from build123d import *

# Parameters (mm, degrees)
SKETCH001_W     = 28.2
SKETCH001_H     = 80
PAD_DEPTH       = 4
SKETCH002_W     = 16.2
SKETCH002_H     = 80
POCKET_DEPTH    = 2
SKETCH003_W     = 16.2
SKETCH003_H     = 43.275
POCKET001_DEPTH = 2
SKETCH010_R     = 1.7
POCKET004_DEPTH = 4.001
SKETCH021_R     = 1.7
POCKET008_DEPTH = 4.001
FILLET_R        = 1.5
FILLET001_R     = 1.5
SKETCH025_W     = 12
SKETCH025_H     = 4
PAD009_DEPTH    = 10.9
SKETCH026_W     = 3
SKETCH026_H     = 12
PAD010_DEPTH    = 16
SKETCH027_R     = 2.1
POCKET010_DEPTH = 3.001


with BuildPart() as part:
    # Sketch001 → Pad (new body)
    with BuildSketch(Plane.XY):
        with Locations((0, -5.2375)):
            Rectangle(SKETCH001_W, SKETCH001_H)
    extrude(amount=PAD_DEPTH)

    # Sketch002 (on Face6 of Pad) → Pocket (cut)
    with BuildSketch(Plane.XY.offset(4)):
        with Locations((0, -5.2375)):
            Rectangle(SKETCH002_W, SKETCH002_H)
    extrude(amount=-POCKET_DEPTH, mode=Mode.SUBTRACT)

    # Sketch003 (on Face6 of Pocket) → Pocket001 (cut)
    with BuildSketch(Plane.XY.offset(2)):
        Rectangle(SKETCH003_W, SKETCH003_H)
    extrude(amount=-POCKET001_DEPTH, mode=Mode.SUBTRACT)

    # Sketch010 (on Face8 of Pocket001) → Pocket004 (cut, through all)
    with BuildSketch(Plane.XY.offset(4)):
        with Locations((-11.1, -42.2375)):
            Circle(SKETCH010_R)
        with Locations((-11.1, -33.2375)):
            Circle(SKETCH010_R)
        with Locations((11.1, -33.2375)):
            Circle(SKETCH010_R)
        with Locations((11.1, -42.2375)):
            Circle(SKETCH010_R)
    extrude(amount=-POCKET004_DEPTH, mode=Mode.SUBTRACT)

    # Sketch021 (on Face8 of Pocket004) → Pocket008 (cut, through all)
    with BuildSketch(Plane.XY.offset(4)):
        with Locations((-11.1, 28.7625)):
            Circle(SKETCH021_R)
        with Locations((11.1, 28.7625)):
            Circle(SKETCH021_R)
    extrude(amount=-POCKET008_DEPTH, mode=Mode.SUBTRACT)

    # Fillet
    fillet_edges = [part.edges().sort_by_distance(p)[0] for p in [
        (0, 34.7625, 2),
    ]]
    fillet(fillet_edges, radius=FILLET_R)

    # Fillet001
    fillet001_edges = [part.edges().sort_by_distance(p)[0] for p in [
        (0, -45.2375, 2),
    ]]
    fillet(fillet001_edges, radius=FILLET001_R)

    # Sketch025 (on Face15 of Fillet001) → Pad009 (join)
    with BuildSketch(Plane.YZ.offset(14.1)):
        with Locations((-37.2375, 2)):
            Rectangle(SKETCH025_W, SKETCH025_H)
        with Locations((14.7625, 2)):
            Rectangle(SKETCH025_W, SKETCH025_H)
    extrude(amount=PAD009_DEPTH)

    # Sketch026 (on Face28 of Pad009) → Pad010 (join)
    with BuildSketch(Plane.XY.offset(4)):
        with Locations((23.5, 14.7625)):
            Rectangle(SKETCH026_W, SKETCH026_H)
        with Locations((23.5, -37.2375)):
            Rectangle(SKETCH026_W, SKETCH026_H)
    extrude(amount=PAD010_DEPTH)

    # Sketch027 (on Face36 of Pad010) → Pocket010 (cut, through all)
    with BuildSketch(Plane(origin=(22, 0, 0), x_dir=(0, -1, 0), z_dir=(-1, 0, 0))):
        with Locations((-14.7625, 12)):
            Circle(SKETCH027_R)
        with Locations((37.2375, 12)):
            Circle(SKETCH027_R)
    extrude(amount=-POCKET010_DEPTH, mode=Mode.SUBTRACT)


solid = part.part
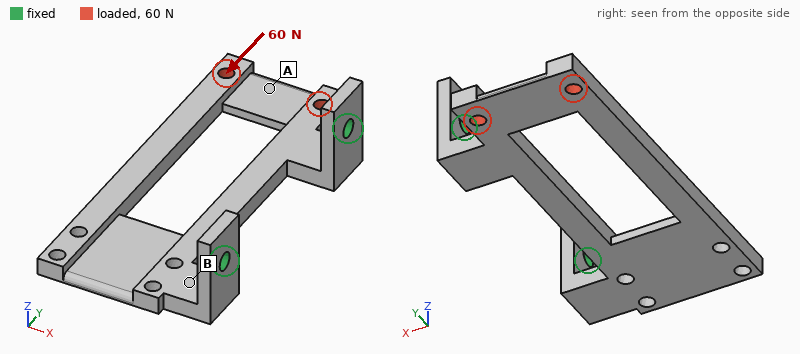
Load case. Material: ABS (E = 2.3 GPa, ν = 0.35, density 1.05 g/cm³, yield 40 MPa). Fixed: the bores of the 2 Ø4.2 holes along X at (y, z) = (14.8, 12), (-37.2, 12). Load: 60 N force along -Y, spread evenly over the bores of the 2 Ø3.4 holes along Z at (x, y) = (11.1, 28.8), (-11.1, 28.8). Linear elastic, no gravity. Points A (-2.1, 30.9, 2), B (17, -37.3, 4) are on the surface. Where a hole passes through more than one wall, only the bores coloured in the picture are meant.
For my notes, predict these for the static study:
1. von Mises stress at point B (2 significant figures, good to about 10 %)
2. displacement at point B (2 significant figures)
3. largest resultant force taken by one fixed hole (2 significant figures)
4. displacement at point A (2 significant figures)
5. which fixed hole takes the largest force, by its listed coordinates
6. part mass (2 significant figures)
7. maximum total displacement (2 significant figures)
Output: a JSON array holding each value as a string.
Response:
["3.1 MPa", "0.12 mm", "41 N", "0.49 mm", "(14.8, 12)", "7.3 g", "0.64 mm"]
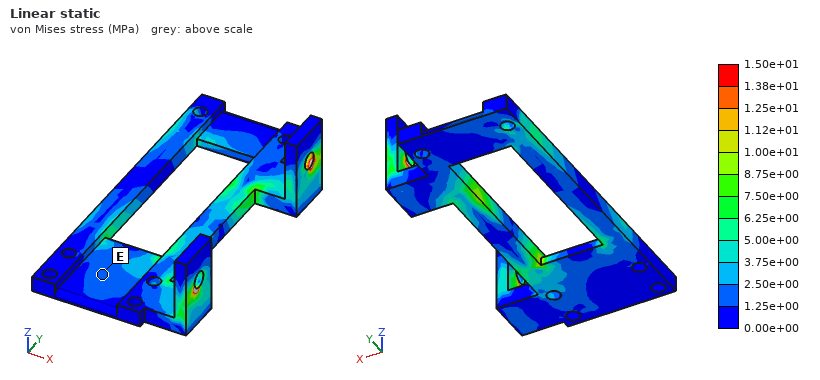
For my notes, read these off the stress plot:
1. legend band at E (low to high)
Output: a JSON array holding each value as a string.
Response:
["1.25e+00 to 2.50e+00 MPa"]
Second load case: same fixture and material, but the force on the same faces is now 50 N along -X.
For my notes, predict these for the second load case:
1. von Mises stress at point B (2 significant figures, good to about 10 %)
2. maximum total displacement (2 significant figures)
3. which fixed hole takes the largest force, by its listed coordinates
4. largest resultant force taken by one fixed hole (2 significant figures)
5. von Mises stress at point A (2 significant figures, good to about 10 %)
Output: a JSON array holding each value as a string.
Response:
["2.5 MPa", "0.98 mm", "(14.8, 12)", "60 N", "2.9 MPa"]
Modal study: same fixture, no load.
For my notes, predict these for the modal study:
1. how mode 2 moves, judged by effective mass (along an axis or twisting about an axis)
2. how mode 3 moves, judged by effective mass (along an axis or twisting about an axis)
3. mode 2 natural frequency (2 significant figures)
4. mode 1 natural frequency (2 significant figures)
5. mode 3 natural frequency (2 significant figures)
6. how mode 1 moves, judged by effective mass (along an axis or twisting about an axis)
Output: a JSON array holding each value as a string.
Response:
["twisting about X", "along Y", "490 Hz", "240 Hz", "860 Hz", "along Z"]
